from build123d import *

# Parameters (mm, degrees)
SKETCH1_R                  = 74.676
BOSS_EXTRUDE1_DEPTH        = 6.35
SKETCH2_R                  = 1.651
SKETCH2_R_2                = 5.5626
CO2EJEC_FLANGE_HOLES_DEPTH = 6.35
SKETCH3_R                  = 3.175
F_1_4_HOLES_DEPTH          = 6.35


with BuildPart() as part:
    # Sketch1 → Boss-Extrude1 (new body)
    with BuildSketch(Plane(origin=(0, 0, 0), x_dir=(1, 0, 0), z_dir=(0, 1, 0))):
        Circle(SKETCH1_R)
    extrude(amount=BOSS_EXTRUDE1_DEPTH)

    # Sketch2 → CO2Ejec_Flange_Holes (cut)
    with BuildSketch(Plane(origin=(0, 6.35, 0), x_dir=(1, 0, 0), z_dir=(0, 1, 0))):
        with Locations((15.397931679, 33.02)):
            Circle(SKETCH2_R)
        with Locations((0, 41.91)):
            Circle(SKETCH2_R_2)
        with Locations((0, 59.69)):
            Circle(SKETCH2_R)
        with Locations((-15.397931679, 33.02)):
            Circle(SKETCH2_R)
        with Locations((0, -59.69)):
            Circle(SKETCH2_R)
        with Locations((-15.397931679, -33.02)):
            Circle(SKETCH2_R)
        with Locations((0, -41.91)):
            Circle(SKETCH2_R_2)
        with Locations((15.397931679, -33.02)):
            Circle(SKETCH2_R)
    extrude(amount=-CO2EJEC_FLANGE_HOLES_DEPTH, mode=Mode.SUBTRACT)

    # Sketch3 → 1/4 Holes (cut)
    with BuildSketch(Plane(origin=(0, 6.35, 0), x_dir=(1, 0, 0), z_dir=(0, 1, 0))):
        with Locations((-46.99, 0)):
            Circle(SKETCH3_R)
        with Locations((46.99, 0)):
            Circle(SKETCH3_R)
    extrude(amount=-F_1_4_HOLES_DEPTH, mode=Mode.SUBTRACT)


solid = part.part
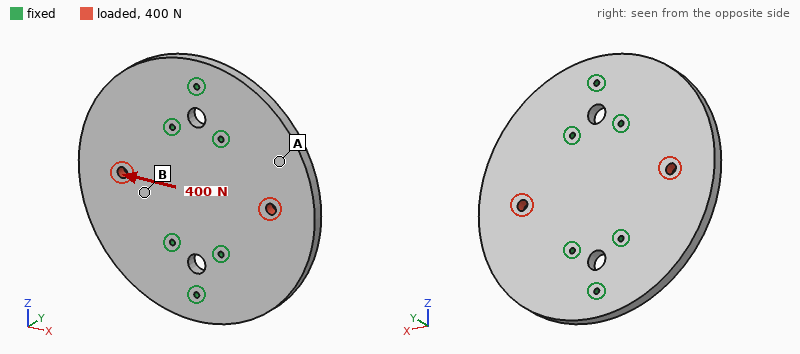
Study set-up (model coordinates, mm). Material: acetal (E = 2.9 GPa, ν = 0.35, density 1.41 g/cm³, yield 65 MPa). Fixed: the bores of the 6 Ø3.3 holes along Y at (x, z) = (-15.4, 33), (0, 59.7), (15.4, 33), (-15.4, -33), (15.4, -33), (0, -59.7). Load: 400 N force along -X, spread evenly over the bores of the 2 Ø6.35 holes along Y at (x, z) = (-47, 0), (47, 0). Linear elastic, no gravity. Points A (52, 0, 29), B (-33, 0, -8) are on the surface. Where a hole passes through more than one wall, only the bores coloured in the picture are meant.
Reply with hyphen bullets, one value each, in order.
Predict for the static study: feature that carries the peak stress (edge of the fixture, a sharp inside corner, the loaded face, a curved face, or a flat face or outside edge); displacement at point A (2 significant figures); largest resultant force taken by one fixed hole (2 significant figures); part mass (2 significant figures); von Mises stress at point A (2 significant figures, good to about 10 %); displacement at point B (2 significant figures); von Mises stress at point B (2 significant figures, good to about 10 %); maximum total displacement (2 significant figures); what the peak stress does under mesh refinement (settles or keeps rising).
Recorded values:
- edge of the fixture
- 5.2 µm
- 86 N
- 150 g
- 0.24 MPa
- 8.8 µm
- 0.61 MPa
- 15 µm
- keeps rising
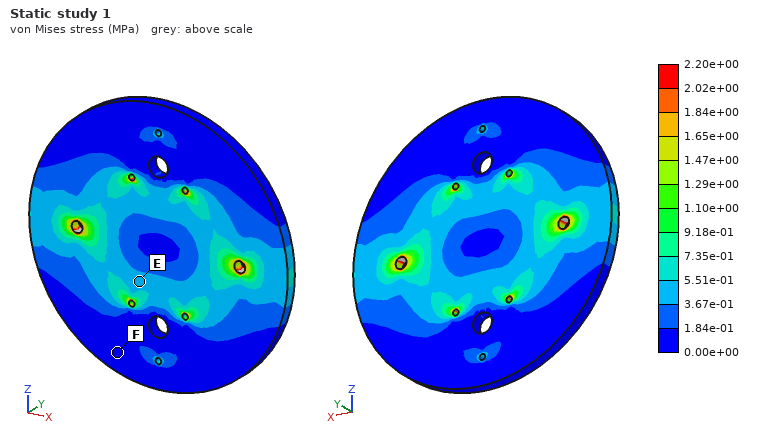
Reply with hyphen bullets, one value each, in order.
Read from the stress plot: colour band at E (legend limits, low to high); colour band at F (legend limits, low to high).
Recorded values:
- 3.67e-01 to 5.51e-01 MPa
- 0.00e+00 to 1.84e-01 MPa
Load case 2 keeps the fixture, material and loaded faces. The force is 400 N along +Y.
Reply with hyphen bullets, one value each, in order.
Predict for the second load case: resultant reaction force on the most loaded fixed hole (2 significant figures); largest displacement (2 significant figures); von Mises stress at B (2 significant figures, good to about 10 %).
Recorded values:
- 140 N
- 1.1 mm
- 4.3 MPa
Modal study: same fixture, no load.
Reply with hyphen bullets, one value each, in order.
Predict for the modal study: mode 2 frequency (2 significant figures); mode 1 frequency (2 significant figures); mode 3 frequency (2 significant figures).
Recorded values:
- 460 Hz
- 460 Hz
- 850 Hz
